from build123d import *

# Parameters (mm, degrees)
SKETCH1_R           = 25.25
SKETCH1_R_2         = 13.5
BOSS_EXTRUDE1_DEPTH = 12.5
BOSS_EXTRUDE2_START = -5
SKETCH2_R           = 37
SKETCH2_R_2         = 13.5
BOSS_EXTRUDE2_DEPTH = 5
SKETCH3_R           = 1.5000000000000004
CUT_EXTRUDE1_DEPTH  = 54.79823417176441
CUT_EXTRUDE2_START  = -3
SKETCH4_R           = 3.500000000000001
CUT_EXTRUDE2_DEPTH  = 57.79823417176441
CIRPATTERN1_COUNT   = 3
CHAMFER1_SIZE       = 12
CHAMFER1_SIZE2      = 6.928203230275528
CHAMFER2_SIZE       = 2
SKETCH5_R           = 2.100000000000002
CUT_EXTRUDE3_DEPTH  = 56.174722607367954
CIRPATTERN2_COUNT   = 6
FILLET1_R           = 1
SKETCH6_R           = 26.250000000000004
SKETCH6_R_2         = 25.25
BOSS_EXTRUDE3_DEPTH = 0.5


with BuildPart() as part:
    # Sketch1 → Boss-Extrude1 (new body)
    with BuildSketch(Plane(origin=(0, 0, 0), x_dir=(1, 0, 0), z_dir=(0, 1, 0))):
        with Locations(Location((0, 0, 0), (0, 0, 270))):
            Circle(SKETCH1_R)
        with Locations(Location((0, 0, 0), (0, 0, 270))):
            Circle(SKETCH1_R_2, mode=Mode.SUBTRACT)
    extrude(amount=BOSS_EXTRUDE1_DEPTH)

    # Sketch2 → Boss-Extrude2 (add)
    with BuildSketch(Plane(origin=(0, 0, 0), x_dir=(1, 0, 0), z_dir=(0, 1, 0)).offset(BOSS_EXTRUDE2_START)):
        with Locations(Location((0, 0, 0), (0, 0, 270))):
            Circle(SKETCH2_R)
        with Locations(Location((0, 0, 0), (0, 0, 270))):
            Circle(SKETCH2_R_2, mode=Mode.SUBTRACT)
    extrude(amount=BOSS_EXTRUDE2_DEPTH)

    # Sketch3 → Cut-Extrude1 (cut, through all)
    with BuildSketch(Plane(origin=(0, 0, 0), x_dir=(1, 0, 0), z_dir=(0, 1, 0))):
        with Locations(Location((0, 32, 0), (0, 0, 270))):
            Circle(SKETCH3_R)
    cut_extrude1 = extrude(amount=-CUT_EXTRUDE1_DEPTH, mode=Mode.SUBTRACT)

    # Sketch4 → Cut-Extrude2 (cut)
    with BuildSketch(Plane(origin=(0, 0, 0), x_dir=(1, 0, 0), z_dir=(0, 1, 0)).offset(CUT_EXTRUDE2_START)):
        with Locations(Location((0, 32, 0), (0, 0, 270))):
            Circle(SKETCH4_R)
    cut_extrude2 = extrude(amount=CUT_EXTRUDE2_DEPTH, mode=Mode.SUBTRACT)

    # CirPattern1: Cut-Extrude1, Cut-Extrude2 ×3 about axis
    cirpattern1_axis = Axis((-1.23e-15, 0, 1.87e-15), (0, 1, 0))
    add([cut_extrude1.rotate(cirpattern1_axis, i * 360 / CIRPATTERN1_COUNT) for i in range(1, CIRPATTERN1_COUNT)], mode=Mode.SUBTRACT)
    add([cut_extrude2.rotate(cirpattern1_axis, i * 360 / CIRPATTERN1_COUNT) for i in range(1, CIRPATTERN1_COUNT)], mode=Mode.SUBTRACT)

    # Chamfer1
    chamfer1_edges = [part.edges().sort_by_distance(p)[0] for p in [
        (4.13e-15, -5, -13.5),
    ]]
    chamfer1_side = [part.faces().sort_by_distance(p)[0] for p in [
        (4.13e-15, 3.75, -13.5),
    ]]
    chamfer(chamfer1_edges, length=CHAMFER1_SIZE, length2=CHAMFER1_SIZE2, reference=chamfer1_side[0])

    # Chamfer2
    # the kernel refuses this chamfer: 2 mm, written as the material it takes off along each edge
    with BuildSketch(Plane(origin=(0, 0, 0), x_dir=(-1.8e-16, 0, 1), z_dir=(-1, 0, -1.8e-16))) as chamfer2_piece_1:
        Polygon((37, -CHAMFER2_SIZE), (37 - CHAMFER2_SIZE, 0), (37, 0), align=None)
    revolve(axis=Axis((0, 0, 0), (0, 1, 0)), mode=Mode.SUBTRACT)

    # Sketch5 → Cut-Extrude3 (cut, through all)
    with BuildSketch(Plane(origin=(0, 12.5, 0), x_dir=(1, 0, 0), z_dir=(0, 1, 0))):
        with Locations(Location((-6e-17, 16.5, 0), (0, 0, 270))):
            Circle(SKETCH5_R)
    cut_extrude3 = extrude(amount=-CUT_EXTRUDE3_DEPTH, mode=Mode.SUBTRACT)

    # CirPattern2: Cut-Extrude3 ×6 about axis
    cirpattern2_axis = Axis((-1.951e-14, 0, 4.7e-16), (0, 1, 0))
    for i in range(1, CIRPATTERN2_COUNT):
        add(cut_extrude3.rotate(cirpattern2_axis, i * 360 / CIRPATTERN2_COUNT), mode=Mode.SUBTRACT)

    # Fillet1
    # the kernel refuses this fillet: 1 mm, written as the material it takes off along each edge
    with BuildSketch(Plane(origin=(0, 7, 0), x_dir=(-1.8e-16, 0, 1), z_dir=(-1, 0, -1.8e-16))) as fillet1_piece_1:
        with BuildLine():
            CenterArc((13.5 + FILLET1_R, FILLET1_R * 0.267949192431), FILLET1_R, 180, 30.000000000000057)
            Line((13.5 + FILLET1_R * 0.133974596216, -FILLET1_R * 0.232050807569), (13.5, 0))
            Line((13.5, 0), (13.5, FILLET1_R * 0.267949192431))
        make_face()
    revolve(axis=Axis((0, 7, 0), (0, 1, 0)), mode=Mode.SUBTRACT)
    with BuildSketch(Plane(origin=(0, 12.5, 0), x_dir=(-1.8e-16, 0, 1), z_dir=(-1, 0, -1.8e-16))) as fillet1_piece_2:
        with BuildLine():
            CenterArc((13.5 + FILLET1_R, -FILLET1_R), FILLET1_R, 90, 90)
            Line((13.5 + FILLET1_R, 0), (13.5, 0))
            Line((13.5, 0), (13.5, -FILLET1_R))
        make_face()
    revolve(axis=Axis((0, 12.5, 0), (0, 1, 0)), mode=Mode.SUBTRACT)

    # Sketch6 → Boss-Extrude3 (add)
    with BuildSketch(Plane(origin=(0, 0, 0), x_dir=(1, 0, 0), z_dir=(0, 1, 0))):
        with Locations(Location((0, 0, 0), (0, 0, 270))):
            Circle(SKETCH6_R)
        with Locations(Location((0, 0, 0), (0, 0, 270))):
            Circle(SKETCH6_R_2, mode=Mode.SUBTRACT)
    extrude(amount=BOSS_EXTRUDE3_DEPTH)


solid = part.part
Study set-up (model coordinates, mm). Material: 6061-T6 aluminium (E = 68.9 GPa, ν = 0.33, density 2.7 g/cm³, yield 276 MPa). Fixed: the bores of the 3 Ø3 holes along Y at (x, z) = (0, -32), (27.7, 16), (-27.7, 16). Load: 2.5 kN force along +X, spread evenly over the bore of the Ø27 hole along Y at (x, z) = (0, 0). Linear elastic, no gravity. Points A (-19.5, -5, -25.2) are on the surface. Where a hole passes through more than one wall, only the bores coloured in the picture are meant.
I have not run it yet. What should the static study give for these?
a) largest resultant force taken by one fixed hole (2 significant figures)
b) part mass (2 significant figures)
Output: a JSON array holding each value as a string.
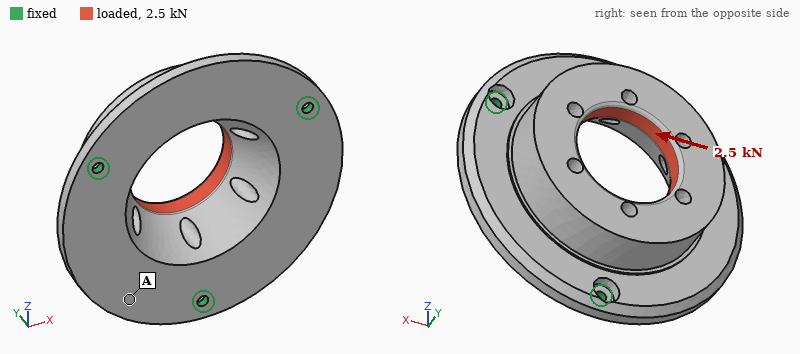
["1.1 kN", "83 g"]
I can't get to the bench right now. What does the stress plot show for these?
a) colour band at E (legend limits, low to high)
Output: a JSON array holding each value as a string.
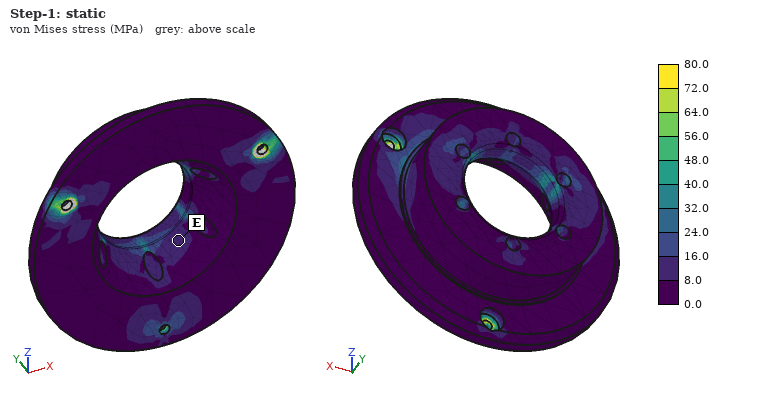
["8.0 to 16.0 MPa"]
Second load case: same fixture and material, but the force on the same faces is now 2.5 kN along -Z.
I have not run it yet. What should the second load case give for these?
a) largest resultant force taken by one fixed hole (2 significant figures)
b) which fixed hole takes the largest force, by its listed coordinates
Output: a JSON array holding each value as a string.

["1.3 kN", "(0, -32)"]
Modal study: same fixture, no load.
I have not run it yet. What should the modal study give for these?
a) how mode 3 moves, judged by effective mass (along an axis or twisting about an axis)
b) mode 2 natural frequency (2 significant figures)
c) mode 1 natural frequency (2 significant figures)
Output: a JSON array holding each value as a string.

["along Y", "6500 Hz", "6400 Hz"]
